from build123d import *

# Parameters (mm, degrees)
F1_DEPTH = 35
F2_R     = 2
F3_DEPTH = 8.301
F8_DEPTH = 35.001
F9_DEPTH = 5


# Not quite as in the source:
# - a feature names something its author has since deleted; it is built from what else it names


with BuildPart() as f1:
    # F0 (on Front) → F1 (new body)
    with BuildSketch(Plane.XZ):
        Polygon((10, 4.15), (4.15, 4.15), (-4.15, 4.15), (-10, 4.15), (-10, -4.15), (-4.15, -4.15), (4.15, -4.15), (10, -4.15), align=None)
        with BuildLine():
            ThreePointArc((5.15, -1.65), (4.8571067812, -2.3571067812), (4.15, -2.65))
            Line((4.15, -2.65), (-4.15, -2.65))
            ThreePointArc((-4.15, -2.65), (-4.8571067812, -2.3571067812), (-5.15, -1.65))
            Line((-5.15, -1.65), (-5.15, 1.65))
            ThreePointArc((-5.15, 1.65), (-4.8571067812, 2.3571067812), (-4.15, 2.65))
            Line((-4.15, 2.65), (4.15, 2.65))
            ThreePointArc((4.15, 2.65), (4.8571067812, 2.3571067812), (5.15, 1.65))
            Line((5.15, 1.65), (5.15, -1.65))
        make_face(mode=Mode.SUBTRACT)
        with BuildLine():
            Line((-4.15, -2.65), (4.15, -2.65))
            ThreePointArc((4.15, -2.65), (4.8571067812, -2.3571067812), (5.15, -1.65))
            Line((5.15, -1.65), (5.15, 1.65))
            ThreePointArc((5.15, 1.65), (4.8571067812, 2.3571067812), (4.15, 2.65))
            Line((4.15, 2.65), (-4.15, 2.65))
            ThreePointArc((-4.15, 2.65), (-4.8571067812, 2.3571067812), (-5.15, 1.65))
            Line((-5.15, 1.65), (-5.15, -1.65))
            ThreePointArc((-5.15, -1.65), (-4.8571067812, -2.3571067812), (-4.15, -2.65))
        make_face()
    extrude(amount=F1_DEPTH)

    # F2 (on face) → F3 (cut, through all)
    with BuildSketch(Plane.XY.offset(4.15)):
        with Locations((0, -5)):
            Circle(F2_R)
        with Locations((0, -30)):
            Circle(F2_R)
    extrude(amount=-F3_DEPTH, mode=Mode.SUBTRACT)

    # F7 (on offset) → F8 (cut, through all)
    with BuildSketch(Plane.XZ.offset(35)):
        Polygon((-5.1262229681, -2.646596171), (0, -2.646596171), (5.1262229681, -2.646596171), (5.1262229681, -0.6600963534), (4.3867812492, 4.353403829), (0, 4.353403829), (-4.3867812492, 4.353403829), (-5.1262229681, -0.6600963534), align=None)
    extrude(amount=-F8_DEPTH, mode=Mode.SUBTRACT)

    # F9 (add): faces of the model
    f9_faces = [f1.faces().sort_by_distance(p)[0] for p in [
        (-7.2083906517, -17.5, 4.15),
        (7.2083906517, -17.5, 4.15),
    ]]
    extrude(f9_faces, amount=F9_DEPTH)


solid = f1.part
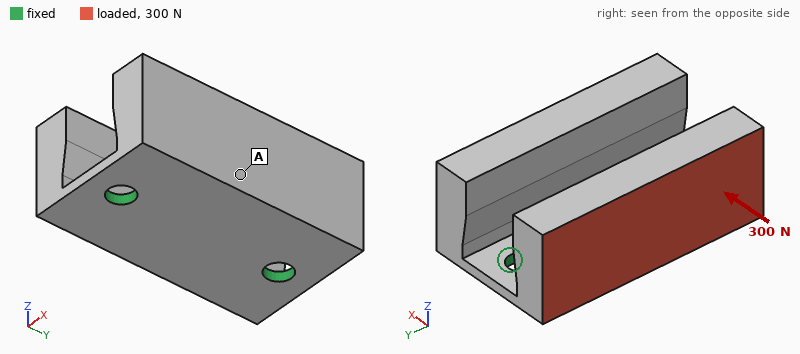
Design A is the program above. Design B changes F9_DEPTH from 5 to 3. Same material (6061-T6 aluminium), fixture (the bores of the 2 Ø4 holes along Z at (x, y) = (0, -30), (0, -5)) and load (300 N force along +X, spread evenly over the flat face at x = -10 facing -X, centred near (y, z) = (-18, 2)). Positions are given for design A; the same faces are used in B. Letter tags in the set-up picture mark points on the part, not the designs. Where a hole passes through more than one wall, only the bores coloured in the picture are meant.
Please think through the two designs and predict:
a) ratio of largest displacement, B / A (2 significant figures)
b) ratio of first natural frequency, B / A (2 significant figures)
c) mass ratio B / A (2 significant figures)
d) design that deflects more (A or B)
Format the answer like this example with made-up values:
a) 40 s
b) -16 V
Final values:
a) 0.73
b) 1.2
c) 0.86
d) A
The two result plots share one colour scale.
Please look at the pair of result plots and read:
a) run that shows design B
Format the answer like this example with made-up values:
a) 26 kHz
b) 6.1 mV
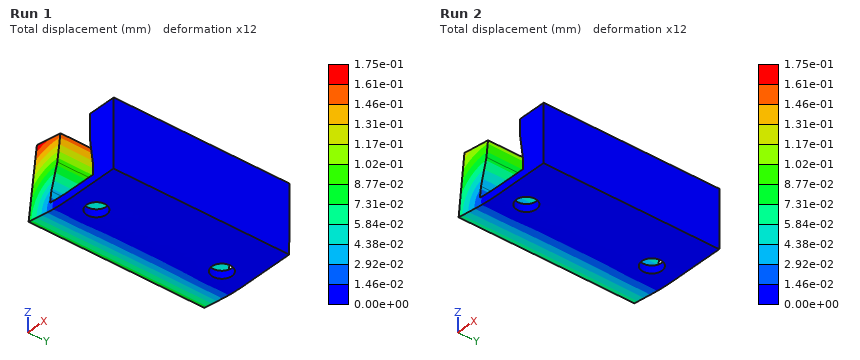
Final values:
a) Run 2
